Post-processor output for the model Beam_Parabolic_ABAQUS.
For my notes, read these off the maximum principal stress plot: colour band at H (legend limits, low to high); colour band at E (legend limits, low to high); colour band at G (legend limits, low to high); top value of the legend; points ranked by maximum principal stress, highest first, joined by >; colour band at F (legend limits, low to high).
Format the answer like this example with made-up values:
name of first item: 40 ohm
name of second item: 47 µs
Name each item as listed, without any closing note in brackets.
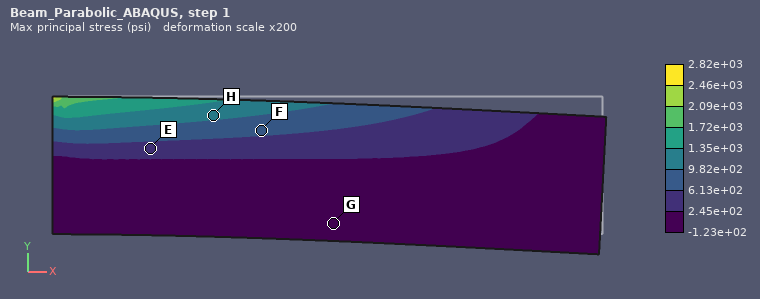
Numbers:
colour band at H: 9.82e+02 to 1.35e+03 psi
colour band at E: 2.45e+02 to 6.13e+02 psi
colour band at G: -1.23e+02 to 2.45e+02 psi
top value of the legend: 2.82e+03 psi
points ranked by maximum principal stress, highest first, joined by >: H > F > E > G
colour band at F: 6.13e+02 to 9.82e+02 psi
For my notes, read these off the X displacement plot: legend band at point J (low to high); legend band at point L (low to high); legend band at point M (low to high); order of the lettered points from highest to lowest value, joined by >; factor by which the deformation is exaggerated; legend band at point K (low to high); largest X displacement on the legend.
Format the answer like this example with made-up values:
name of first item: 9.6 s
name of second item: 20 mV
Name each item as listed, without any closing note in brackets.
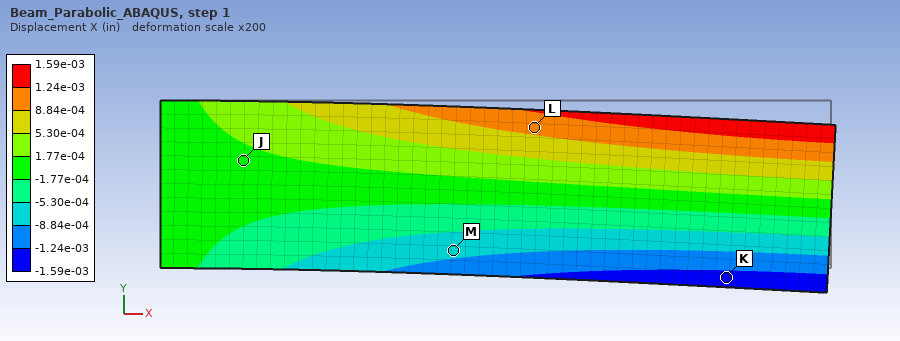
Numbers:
legend band at point J: -1.77e-04 to 1.77e-04 in
legend band at point L: 8.84e-04 to 1.24e-03 in
legend band at point M: -8.84e-04 to -5.30e-04 in
order of the lettered points from highest to lowest value, joined by >: L > J > M > K
factor by which the deformation is exaggerated: 200
legend band at point K: -1.59e-03 to -1.24e-03 in
largest X displacement on the legend: 1.59e-03 in
